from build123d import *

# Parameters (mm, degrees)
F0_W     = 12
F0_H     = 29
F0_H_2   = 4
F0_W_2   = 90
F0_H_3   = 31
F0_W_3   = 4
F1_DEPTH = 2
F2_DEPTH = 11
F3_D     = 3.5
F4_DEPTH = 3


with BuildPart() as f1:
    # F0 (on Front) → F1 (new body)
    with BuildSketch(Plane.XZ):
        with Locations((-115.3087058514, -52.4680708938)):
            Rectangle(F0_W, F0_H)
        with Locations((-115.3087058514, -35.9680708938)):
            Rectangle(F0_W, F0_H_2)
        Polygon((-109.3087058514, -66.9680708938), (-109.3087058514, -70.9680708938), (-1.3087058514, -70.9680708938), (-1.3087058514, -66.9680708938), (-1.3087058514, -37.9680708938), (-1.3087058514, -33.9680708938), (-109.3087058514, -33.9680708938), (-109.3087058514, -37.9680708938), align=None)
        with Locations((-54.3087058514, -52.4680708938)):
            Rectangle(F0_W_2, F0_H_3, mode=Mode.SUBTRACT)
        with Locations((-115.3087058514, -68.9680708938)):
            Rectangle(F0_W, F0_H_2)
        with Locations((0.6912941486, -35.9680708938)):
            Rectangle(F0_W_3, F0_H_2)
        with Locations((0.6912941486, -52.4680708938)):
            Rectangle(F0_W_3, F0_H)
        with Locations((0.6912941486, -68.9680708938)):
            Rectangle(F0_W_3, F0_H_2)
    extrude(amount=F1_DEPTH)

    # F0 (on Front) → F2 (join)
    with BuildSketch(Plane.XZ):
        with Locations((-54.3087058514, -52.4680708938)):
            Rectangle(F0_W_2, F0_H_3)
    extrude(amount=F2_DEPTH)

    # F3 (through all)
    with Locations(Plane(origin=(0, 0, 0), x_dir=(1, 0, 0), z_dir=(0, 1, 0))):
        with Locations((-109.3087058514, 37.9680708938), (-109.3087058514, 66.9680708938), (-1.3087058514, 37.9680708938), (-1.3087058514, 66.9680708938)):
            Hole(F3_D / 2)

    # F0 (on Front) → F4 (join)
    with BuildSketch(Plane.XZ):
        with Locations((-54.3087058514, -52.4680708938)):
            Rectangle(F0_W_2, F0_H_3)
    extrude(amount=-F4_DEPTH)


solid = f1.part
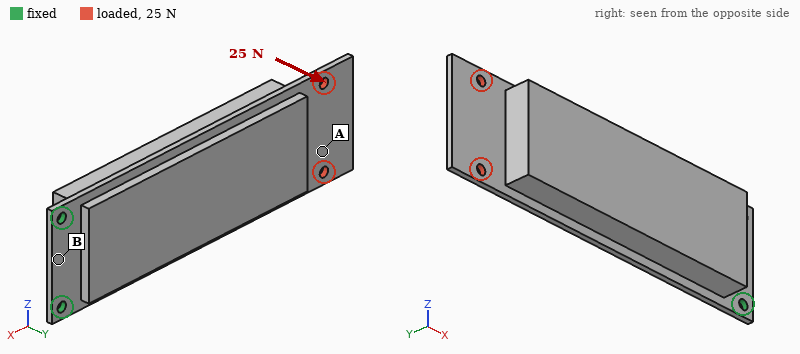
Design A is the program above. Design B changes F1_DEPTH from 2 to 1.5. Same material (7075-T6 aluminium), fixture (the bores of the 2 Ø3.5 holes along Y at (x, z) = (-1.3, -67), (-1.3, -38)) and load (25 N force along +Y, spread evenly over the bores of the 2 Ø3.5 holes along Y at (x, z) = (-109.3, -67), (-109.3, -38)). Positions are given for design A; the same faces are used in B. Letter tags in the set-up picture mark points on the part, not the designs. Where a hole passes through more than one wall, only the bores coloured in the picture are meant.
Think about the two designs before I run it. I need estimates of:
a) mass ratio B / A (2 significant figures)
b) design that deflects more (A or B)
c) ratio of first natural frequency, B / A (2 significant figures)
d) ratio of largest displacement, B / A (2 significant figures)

0.98
B
0.68
2.2
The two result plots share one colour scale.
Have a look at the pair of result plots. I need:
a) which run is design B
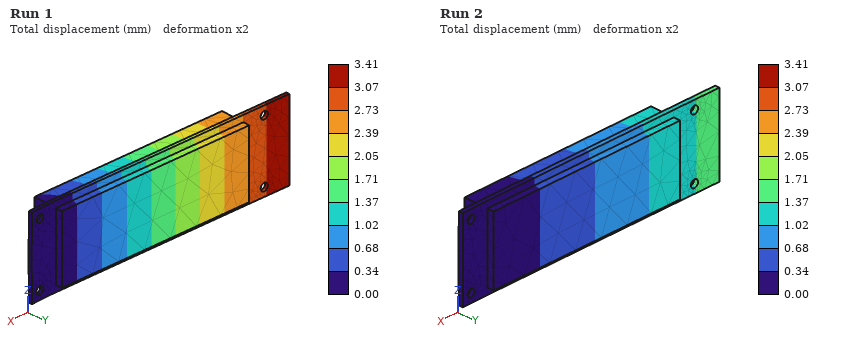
Run 1
